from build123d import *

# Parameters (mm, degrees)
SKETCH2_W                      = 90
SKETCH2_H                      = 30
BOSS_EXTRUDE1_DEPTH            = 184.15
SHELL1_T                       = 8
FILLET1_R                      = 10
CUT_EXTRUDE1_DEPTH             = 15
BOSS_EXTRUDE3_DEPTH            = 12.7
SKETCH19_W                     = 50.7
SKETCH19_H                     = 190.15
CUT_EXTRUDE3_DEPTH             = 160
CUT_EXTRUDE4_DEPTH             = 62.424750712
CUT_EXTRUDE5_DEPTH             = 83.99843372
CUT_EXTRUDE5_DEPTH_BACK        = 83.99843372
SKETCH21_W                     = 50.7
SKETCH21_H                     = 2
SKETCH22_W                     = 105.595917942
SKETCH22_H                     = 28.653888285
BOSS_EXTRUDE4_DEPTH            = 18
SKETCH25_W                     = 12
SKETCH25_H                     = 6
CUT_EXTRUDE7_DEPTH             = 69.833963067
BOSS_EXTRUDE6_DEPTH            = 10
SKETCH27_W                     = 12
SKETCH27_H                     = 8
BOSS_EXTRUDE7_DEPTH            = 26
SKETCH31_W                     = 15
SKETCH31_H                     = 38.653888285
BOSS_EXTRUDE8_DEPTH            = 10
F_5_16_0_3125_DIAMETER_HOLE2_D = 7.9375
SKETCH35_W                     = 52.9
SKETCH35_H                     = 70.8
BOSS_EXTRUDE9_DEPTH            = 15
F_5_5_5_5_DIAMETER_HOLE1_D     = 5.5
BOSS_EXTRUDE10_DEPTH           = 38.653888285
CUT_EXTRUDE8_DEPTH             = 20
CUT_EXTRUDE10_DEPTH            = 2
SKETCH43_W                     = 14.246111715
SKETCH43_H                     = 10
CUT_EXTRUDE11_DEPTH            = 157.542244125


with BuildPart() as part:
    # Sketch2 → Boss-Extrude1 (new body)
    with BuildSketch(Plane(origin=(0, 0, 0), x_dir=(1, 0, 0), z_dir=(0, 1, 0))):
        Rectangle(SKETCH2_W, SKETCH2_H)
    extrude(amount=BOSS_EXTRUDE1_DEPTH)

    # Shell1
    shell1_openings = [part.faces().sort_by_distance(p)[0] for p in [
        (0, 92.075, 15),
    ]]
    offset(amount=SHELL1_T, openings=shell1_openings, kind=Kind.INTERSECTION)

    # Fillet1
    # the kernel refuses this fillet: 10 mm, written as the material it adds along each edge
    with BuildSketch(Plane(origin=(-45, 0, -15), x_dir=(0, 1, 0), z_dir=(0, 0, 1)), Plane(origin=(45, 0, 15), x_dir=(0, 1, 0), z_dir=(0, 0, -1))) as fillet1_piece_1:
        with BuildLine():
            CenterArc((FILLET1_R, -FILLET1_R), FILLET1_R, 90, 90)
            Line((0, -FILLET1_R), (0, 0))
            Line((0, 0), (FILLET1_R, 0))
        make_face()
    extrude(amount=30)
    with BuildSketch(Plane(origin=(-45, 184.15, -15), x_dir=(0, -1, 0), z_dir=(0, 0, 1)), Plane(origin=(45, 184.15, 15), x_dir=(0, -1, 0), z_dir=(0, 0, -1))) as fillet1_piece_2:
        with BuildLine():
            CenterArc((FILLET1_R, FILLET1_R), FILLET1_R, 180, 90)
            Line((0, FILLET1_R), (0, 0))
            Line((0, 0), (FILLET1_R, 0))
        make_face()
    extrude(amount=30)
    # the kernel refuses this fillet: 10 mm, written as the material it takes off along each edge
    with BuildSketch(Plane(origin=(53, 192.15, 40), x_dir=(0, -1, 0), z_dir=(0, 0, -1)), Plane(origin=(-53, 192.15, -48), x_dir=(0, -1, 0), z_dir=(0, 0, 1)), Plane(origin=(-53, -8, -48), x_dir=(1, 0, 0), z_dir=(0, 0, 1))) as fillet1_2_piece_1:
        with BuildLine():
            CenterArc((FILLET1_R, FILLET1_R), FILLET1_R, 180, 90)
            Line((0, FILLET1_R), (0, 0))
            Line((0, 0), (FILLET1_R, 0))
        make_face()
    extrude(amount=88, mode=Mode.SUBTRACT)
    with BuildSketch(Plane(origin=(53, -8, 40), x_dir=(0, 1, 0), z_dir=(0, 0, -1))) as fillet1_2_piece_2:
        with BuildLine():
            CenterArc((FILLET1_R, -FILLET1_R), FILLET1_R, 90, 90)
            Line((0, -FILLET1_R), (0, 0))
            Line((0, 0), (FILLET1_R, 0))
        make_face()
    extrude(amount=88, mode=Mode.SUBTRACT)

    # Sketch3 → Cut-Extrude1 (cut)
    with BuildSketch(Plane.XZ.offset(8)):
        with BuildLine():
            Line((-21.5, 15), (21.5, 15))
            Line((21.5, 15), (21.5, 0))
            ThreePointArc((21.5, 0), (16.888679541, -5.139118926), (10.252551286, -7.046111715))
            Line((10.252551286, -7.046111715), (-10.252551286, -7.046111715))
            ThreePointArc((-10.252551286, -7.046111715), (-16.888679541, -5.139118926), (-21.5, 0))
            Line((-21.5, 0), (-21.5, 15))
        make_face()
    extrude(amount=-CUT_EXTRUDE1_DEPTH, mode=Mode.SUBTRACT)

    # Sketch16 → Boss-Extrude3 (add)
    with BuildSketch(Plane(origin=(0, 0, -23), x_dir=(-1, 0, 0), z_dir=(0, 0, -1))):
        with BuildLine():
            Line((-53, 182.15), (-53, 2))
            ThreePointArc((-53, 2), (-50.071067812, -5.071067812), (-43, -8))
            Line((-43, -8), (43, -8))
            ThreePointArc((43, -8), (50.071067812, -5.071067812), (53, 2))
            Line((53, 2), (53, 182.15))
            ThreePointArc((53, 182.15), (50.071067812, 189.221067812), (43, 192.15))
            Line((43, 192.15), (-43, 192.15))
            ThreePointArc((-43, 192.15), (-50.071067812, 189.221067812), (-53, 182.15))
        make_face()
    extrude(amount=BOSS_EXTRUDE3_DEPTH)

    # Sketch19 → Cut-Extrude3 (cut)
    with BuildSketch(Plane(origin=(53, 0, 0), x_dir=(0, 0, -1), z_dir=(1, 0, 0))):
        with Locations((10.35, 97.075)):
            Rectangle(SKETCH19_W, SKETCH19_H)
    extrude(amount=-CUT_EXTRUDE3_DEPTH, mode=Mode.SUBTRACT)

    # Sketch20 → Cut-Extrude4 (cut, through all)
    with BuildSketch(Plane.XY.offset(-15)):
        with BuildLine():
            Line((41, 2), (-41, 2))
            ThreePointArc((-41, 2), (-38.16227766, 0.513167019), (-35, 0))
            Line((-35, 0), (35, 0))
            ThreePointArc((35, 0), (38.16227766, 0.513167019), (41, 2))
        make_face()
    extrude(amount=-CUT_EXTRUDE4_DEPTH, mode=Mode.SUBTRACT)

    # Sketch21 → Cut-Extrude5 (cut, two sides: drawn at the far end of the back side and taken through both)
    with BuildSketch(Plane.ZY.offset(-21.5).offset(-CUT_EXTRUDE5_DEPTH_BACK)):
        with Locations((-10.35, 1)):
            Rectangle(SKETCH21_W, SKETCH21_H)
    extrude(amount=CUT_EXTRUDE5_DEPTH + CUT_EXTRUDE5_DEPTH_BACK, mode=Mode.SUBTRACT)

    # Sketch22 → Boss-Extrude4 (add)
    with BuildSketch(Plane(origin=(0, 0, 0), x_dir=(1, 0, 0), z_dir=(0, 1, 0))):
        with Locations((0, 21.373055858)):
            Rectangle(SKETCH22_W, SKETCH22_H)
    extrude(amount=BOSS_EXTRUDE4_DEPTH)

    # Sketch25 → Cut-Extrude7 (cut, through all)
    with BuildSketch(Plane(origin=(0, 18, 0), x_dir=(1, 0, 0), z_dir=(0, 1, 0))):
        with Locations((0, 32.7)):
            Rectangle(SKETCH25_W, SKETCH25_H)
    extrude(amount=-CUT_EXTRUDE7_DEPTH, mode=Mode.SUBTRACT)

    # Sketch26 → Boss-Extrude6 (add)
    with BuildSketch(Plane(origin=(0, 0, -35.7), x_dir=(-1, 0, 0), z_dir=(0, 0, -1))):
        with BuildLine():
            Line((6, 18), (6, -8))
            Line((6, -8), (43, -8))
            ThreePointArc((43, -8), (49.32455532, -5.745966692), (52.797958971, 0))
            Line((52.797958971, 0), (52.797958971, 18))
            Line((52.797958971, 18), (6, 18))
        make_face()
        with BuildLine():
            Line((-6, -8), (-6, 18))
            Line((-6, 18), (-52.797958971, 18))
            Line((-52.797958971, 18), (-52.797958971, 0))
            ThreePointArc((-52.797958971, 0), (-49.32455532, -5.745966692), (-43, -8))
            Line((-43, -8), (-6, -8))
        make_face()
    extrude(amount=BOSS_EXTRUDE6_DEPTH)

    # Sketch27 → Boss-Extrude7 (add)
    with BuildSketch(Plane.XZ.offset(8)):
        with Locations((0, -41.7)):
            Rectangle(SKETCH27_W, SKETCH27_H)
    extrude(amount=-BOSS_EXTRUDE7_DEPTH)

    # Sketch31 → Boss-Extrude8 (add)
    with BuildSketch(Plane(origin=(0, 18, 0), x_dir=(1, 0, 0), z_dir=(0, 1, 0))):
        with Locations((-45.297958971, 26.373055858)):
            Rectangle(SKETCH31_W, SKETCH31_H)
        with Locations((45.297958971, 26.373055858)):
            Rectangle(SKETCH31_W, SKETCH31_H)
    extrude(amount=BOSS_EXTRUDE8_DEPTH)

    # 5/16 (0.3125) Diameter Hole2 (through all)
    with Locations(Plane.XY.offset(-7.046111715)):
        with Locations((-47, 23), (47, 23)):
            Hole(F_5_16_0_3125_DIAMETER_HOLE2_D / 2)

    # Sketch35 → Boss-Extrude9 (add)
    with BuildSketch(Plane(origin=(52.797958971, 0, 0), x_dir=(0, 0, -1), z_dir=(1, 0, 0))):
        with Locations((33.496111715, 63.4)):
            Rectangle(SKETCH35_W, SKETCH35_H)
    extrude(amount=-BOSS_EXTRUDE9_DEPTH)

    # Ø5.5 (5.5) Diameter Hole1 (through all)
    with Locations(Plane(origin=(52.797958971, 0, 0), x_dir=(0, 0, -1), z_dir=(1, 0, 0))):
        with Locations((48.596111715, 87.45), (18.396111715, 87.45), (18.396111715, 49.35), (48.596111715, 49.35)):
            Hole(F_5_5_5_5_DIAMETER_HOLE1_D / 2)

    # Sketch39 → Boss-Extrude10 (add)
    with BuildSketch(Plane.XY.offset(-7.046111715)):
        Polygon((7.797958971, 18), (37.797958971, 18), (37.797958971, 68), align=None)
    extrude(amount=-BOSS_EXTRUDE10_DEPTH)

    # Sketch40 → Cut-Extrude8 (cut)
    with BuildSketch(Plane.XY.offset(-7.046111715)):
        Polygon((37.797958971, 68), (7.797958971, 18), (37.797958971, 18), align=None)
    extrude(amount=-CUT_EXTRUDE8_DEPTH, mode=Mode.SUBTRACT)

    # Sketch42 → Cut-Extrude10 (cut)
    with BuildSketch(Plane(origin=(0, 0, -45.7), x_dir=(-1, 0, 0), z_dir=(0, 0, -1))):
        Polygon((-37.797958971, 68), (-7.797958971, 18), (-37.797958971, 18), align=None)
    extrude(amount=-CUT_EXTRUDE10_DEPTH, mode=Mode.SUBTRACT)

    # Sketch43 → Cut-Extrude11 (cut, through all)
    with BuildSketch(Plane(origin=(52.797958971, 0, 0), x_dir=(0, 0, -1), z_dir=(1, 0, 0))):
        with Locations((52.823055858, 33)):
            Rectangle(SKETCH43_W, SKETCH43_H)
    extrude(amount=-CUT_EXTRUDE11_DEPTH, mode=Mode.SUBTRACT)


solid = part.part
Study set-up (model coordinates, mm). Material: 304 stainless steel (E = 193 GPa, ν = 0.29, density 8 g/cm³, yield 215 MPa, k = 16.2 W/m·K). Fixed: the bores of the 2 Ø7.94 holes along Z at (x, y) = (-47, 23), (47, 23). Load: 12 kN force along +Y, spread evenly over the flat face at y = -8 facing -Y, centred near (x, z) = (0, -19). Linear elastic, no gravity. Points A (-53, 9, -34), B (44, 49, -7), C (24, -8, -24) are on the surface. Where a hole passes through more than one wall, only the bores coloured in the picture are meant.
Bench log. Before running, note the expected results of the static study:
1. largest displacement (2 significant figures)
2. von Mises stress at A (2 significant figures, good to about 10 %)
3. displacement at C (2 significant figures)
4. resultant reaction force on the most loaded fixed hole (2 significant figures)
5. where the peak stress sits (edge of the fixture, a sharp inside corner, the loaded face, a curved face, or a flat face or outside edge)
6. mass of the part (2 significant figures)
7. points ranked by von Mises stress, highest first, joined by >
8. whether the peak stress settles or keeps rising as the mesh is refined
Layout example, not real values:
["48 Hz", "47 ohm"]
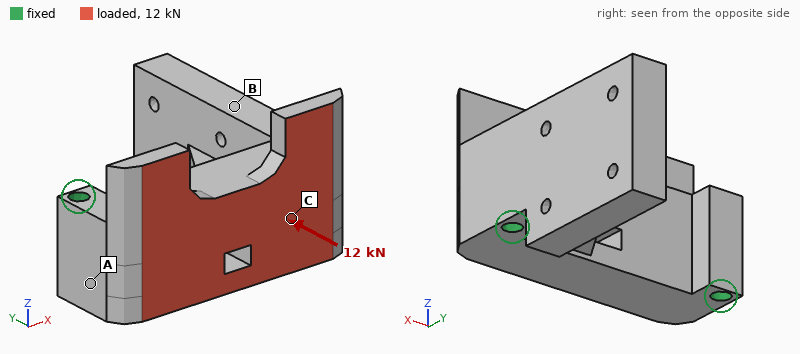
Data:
["24 µm", "7.1 MPa", "4.1 µm", "7.6 kN", "edge of the fixture", "1.5 kg", "C > A > B", "keeps rising"]
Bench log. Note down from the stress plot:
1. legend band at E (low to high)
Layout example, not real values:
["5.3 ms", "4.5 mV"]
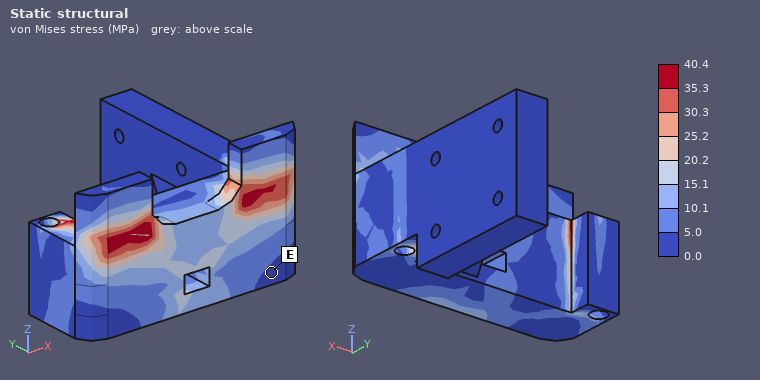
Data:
["0.0 to 5.0 MPa"]
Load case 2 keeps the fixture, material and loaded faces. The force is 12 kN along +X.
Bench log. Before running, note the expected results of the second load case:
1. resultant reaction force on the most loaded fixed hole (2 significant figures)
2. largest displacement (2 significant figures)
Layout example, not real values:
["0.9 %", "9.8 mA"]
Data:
["7.3 kN", "8.1 µm"]
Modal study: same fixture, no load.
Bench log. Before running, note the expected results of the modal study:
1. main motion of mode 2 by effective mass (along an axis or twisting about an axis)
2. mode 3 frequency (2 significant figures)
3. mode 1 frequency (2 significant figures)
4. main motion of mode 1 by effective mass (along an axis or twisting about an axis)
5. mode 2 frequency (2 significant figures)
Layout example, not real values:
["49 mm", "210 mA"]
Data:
["along Z", "5900 Hz", "3000 Hz", "along X", "4300 Hz"]
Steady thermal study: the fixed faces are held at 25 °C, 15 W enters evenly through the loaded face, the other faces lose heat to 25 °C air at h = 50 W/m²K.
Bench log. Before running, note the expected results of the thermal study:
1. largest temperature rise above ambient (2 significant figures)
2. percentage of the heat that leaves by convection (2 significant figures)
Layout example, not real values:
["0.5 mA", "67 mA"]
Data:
["14 K", "38 %"]
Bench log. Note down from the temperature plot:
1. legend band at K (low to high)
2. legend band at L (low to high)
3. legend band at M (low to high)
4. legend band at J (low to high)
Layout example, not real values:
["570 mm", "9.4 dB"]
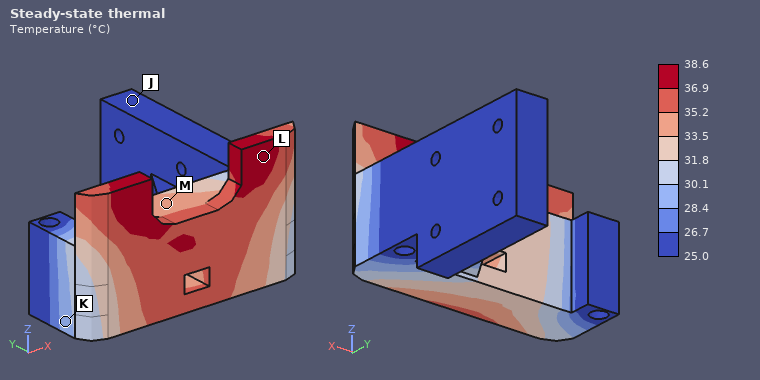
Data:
["28.4 to 30.1 °C", "36.9 to 38.6 °C", "33.5 to 35.2 °C", "25.0 to 26.7 °C"]
